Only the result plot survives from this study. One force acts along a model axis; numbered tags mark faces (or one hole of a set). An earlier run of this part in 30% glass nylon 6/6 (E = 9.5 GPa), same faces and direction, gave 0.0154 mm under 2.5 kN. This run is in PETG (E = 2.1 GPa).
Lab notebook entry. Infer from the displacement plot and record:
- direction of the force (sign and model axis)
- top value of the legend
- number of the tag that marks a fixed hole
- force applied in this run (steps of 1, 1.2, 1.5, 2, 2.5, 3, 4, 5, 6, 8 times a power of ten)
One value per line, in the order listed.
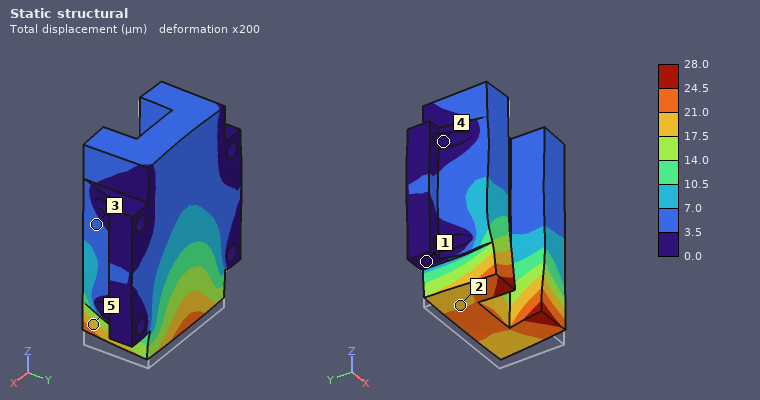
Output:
+Z
28.0 µm
4
1 kN
